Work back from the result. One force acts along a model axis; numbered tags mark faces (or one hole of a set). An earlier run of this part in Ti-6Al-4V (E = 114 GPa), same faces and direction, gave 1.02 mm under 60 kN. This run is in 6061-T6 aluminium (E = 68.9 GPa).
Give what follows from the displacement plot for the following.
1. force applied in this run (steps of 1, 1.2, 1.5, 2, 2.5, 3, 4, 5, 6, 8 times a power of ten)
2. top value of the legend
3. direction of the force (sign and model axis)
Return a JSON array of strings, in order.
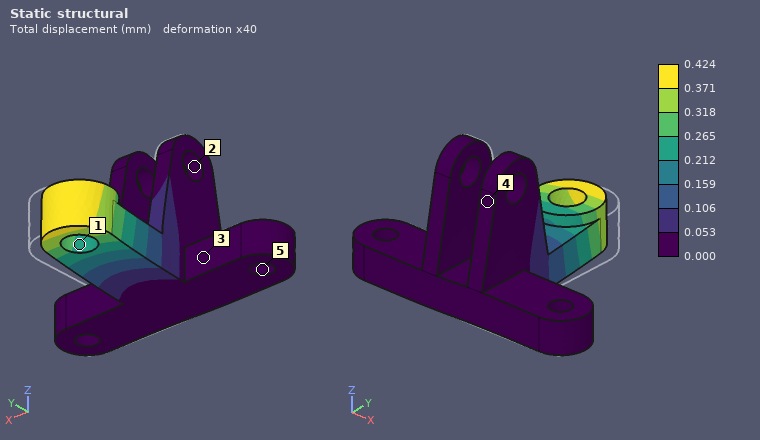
["15 kN", "0.424 mm", "-X"]
